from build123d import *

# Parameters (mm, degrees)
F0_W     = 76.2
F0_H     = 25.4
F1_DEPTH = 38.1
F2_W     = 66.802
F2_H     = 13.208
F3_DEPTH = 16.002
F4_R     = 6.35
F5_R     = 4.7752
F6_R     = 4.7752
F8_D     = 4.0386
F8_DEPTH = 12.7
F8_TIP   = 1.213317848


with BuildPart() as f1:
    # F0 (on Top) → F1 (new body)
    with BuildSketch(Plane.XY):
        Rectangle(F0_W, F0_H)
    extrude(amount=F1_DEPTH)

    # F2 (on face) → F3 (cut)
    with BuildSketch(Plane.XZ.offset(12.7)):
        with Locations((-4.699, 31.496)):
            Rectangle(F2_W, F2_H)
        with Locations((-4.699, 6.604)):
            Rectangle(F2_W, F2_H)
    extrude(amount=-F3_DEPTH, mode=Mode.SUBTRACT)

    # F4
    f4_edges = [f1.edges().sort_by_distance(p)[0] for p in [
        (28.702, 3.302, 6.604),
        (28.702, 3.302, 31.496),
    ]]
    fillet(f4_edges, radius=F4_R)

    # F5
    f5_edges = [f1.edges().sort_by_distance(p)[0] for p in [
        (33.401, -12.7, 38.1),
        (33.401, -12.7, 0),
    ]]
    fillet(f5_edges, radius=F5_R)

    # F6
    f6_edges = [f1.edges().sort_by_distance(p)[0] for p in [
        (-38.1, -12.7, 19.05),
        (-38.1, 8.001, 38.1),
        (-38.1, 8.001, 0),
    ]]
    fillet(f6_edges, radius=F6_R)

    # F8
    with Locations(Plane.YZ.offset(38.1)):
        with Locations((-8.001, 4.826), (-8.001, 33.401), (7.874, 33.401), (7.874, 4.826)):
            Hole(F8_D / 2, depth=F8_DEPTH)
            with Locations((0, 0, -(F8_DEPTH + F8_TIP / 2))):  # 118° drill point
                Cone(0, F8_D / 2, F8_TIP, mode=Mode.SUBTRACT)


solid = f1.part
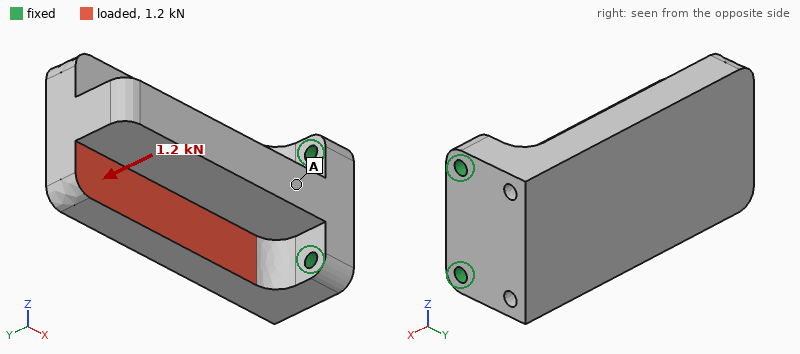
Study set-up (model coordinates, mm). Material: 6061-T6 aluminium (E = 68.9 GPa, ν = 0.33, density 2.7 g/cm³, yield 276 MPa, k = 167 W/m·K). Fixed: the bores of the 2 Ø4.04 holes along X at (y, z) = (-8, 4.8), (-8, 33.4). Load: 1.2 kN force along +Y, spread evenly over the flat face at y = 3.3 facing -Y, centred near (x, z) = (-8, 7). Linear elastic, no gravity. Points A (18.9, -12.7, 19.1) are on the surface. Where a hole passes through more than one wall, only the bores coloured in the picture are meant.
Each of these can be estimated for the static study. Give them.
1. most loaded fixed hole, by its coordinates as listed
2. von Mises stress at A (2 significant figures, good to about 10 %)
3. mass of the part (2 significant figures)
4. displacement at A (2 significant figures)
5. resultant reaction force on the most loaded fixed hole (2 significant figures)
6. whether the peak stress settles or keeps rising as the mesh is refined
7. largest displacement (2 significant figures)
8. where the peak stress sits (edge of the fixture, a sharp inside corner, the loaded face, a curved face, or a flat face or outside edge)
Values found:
(-8, 4.8)
24 MPa
120 g
0.049 mm
1.2 kN
keeps rising
0.25 mm
edge of the fixture
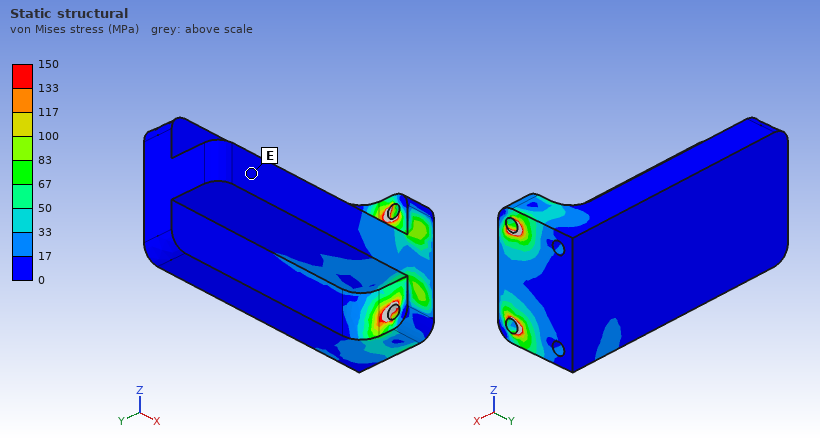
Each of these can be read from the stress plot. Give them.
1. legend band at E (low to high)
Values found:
0 to 17 MPa
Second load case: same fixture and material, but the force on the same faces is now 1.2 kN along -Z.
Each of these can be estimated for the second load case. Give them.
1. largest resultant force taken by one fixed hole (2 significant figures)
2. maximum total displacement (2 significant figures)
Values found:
1.9 kN
79 µm
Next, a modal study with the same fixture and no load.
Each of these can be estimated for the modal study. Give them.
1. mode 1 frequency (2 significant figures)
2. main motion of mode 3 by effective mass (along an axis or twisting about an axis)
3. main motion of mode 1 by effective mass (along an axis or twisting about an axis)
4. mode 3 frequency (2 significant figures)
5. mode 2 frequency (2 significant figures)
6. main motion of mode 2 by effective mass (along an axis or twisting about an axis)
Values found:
1400 Hz
twisting about X
along Y
6300 Hz
2600 Hz
along Z
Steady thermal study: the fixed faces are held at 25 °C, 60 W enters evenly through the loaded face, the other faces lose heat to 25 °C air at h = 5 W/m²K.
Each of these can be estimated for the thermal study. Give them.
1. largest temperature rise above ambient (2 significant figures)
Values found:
42 K
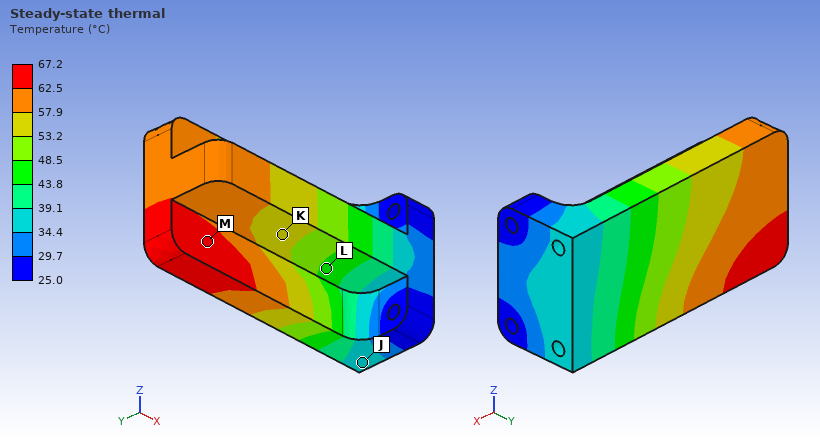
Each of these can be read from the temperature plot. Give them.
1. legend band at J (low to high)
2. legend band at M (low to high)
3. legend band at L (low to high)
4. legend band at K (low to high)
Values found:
34.4 to 39.1 °C
62.5 to 67.2 °C
43.8 to 48.5 °C
53.2 to 57.9 °C
